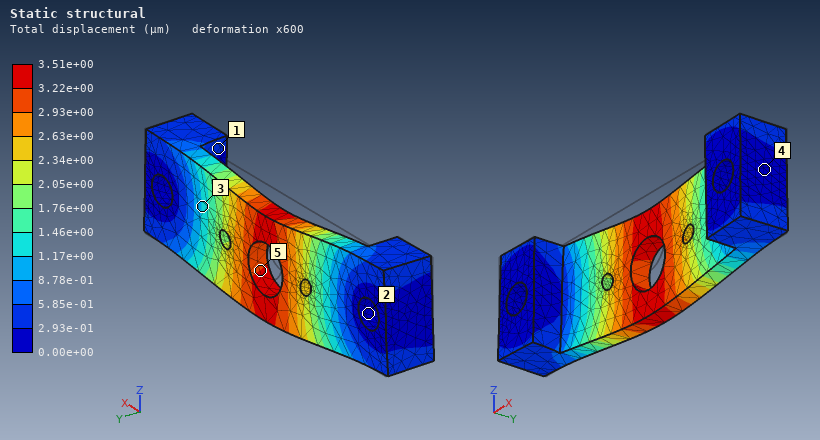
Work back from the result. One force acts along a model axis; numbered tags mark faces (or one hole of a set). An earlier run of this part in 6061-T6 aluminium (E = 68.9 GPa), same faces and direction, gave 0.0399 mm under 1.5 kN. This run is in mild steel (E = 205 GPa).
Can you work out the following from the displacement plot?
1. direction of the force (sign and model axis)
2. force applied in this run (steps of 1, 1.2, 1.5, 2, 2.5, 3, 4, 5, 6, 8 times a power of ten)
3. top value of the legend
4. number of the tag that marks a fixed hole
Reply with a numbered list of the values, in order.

1. -Z
2. 400 N
3. 3.51e+00 µm
4. 2
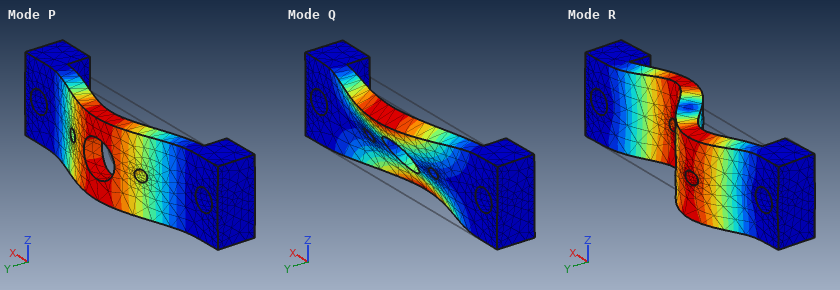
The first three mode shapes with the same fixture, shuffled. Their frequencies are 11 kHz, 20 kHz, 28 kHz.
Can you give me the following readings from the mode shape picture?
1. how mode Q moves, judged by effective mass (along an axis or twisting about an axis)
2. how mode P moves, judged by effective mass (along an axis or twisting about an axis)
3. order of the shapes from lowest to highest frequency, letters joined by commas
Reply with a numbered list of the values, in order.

1. twisting about X
2. along Y
3. P, Q, R
